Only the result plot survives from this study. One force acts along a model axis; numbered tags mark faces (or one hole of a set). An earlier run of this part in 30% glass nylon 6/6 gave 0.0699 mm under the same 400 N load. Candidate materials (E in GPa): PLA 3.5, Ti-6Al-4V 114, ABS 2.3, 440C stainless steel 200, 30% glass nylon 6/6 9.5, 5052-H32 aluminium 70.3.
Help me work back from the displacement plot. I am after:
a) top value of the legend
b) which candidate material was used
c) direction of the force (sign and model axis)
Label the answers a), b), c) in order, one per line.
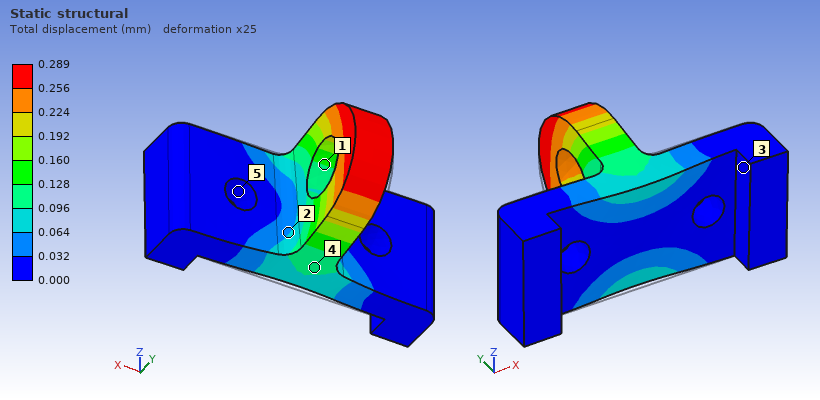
a) 0.289 mm
b) ABS
c) +Z
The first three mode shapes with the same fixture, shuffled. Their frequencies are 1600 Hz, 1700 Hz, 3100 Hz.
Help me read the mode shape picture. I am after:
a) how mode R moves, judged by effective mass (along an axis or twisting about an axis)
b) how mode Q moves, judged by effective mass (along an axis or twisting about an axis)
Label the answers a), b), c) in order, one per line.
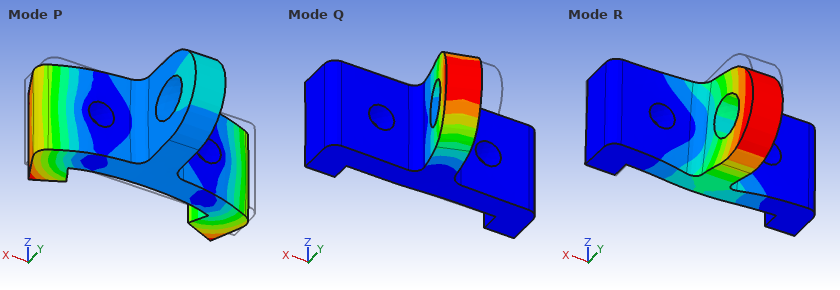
a) along Z
b) along X
